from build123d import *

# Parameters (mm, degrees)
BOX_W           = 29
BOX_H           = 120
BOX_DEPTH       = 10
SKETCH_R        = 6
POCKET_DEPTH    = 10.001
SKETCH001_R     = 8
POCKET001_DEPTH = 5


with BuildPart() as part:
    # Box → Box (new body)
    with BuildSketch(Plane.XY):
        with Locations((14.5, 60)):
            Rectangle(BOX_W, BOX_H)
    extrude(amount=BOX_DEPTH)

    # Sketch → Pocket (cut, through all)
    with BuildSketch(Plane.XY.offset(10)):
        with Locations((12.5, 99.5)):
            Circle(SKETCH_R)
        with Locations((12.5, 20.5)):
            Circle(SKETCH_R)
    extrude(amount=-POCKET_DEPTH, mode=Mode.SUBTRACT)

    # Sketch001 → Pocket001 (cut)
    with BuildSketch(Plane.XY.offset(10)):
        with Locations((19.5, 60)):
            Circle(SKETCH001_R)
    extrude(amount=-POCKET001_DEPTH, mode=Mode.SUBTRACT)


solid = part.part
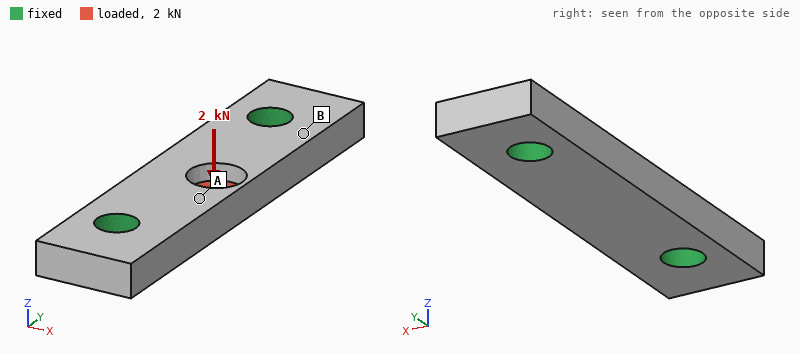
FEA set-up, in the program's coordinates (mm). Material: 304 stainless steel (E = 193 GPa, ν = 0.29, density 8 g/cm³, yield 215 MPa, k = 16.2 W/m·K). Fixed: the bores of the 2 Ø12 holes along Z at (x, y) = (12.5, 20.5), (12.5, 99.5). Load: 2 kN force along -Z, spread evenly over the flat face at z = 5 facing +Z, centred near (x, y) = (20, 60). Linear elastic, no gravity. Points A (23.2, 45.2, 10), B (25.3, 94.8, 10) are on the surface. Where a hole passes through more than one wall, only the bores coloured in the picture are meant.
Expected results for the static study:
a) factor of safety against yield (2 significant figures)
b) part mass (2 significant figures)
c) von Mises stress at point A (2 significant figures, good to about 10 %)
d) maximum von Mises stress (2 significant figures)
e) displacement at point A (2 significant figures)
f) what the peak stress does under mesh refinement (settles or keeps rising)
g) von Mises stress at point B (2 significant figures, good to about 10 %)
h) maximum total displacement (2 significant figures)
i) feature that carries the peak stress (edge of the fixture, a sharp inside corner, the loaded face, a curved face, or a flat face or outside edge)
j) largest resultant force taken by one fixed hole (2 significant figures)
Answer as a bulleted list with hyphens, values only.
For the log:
- 1.7
- 250 g
- 9.3 MPa
- 120 MPa
- 9.8 µm
- settles
- 25 MPa
- 17 µm
- a curved face
- 1.1 kN
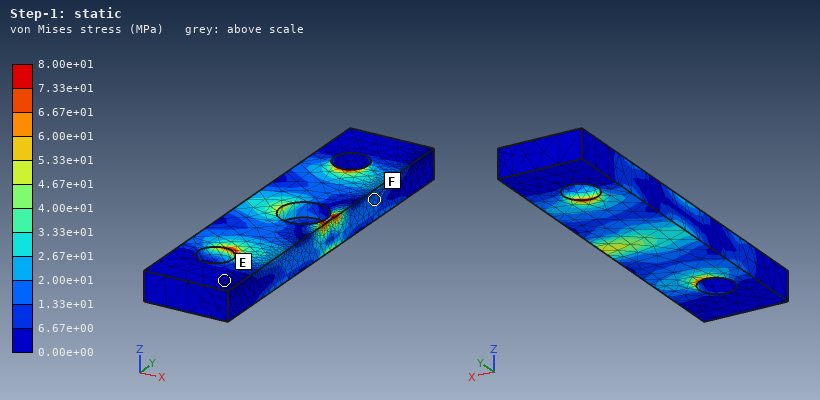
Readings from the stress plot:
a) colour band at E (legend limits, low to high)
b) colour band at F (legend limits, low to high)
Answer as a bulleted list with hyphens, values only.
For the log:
- 0.00e+00 to 6.67e+00 MPa
- 1.33e+01 to 2.00e+01 MPa
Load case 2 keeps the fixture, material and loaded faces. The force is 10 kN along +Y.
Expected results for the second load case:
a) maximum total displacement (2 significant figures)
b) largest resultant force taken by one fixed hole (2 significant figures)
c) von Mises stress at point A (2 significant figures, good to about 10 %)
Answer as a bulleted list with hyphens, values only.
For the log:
- 7.4 µm
- 5.1 kN
- 18 MPa
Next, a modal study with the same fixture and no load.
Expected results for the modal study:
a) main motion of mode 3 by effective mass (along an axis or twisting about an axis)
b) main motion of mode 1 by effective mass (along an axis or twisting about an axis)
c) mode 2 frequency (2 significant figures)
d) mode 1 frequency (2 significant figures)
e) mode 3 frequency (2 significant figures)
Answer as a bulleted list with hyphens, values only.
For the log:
- along X
- along Z
- 13 kHz
- 8600 Hz
- 14 kHz
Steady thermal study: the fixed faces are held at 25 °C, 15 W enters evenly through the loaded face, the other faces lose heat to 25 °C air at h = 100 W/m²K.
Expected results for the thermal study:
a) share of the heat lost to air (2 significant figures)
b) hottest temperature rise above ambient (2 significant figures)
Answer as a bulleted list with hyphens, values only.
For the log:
- 58 %
- 56 K
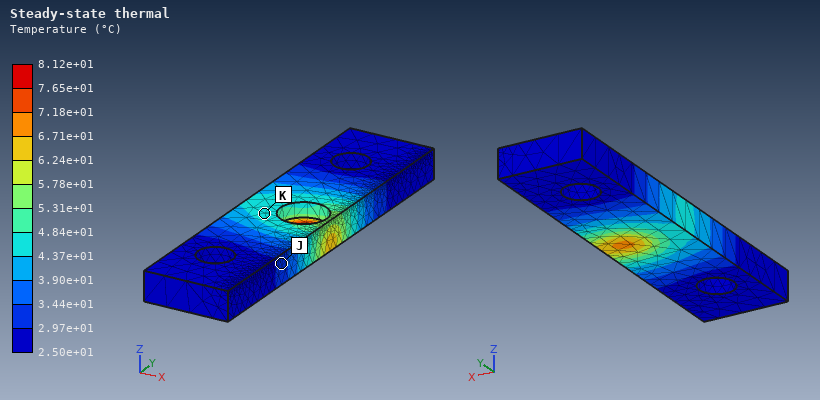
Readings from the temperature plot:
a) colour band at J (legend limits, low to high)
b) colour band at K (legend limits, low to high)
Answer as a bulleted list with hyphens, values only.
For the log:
- 2.97e+01 to 3.44e+01 °C
- 4.37e+01 to 4.84e+01 °C
